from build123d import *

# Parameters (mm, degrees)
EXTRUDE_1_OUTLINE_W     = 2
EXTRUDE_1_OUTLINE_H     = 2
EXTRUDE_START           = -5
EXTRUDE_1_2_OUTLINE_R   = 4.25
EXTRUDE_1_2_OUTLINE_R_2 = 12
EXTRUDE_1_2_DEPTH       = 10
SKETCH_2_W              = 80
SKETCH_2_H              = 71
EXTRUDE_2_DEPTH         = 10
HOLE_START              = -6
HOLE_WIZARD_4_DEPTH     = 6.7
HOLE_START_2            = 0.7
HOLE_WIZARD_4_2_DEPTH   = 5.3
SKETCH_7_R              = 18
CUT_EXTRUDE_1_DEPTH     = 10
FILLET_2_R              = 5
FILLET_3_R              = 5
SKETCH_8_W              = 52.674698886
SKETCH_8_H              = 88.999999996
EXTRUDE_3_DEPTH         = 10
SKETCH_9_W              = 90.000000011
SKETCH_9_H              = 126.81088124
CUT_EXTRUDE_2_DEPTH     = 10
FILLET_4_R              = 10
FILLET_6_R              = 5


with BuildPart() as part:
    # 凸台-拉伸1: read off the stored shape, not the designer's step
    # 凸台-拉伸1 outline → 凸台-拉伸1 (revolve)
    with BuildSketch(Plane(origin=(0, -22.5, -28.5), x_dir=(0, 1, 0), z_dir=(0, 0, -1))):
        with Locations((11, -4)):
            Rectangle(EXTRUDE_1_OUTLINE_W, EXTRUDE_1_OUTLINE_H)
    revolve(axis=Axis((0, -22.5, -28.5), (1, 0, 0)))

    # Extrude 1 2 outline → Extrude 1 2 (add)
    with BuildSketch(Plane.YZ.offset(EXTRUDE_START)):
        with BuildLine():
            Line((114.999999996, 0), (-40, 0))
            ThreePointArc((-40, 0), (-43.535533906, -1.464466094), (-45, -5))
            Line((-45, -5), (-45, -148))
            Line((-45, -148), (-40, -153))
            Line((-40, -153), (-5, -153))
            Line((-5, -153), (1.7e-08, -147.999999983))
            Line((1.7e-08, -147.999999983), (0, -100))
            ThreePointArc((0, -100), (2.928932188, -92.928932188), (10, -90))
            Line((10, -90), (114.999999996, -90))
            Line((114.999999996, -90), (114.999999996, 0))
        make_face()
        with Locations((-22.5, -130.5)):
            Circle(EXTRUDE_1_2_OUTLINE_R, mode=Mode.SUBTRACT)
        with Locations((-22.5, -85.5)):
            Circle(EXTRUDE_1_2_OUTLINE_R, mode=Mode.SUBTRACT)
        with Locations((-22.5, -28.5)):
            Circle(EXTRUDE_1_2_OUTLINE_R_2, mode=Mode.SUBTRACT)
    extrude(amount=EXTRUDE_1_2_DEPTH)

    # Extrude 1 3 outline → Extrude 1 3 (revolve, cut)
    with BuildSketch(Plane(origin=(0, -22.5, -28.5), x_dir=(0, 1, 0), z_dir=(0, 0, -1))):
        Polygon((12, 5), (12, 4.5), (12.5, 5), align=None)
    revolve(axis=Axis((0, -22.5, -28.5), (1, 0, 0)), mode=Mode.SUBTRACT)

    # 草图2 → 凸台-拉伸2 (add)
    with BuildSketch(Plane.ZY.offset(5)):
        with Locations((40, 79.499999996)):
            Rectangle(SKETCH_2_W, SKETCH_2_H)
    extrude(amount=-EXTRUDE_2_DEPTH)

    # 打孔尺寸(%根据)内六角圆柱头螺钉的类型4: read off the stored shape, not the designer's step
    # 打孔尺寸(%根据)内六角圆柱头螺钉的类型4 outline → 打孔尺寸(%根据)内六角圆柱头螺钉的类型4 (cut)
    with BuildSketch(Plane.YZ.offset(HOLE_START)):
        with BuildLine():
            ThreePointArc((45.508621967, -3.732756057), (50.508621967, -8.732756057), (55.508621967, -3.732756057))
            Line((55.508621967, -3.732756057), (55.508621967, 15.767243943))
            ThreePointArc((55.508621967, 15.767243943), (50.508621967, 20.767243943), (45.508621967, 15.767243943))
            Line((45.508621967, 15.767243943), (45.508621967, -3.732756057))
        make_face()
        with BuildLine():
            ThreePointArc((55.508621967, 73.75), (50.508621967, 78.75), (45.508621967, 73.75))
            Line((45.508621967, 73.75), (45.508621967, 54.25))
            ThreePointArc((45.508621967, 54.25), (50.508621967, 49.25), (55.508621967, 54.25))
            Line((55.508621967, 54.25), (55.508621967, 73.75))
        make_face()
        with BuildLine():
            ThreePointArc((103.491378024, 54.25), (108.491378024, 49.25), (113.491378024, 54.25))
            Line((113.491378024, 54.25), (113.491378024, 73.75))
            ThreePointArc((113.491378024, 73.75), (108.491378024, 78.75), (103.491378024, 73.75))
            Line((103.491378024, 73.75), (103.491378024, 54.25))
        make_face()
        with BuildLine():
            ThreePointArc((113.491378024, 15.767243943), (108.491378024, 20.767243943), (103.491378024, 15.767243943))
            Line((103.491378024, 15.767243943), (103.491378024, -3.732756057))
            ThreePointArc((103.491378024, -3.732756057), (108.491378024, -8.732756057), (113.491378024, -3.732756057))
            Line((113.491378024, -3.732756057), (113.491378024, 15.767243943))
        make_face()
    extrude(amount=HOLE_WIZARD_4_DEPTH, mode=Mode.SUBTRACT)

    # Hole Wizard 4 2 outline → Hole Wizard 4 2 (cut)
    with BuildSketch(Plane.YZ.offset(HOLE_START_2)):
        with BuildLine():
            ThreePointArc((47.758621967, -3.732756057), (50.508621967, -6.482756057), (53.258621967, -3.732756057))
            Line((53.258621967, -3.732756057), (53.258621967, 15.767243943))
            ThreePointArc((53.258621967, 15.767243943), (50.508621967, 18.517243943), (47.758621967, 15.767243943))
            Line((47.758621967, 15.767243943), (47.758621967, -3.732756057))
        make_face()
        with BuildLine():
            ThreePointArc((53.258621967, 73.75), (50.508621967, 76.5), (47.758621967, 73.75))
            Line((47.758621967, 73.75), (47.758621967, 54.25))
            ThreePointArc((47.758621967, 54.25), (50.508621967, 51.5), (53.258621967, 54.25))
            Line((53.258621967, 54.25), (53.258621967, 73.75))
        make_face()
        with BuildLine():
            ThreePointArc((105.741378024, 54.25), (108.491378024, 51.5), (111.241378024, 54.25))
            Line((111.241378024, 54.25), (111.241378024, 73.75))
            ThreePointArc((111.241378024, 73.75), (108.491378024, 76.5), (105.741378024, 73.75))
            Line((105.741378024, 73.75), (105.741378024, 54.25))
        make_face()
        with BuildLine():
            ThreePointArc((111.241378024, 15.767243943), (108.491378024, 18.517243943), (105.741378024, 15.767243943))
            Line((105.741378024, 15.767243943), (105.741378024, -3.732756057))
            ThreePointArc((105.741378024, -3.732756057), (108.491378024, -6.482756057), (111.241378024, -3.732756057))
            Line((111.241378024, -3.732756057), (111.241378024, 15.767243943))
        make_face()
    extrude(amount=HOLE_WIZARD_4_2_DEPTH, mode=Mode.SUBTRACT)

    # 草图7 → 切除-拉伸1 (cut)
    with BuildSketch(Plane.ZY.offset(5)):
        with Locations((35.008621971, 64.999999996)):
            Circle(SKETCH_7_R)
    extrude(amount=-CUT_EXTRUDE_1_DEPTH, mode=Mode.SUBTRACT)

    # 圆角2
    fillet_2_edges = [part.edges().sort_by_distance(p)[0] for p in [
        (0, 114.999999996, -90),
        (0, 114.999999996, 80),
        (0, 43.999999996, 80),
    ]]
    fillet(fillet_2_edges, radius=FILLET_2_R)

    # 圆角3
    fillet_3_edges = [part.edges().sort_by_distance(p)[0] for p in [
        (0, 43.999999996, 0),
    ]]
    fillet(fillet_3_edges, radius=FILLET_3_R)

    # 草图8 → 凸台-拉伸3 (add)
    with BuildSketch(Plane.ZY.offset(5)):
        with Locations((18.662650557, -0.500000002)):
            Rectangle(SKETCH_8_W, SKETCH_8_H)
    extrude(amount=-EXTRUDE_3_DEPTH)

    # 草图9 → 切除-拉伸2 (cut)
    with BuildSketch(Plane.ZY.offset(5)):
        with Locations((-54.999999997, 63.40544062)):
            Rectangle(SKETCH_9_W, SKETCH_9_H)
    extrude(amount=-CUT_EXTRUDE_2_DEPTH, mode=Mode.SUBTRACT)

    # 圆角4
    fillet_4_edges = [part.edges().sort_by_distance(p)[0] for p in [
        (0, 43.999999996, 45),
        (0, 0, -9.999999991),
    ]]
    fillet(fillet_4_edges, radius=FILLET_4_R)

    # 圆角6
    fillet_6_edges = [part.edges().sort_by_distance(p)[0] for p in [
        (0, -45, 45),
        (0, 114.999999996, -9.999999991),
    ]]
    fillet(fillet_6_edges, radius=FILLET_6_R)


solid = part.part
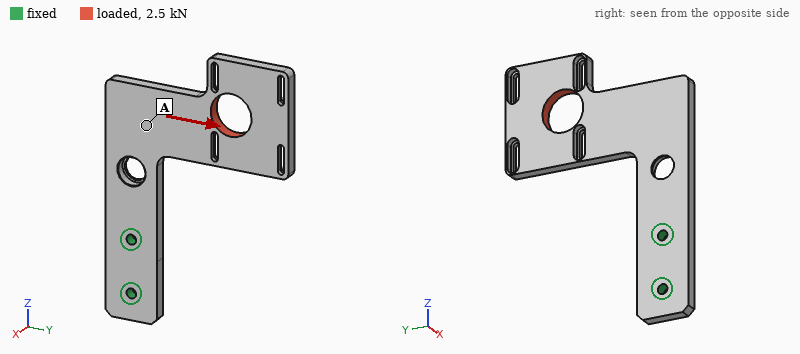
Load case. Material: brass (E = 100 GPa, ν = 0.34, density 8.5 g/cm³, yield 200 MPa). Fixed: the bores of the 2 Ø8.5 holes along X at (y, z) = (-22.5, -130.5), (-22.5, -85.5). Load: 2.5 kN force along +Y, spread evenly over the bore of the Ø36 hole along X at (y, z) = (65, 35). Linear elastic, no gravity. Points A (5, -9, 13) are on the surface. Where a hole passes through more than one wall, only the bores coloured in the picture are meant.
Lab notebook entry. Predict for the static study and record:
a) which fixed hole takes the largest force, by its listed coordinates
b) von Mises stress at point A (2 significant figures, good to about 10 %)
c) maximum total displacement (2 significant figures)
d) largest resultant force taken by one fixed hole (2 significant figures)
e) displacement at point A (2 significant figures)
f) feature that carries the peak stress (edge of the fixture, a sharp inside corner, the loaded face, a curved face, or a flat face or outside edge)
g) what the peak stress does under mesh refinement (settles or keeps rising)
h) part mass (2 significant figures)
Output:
(-22.5, -85.5)
13 MPa
0.69 mm
7.4 kN
0.26 mm
edge of the fixture
keeps rising
1.3 kg
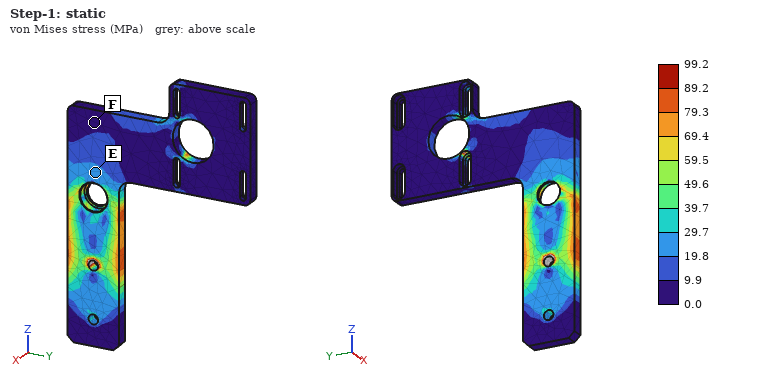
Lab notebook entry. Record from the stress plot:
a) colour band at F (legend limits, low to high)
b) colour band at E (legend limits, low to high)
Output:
0.0 to 9.9 MPa
19.8 to 29.7 MPa
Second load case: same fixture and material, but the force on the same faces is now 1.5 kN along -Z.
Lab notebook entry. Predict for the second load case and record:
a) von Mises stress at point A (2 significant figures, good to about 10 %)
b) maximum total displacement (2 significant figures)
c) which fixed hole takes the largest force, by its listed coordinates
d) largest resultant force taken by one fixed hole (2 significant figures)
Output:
11 MPa
0.43 mm
(-22.5, -85.5)
2.5 kN
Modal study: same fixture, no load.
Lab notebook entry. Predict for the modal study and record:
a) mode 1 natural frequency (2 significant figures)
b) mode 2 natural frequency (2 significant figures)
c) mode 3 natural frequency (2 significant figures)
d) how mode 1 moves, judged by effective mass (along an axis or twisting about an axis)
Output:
100 Hz
300 Hz
380 Hz
along X
